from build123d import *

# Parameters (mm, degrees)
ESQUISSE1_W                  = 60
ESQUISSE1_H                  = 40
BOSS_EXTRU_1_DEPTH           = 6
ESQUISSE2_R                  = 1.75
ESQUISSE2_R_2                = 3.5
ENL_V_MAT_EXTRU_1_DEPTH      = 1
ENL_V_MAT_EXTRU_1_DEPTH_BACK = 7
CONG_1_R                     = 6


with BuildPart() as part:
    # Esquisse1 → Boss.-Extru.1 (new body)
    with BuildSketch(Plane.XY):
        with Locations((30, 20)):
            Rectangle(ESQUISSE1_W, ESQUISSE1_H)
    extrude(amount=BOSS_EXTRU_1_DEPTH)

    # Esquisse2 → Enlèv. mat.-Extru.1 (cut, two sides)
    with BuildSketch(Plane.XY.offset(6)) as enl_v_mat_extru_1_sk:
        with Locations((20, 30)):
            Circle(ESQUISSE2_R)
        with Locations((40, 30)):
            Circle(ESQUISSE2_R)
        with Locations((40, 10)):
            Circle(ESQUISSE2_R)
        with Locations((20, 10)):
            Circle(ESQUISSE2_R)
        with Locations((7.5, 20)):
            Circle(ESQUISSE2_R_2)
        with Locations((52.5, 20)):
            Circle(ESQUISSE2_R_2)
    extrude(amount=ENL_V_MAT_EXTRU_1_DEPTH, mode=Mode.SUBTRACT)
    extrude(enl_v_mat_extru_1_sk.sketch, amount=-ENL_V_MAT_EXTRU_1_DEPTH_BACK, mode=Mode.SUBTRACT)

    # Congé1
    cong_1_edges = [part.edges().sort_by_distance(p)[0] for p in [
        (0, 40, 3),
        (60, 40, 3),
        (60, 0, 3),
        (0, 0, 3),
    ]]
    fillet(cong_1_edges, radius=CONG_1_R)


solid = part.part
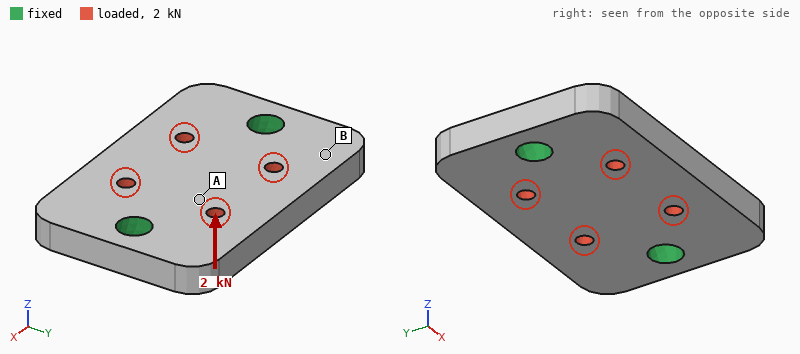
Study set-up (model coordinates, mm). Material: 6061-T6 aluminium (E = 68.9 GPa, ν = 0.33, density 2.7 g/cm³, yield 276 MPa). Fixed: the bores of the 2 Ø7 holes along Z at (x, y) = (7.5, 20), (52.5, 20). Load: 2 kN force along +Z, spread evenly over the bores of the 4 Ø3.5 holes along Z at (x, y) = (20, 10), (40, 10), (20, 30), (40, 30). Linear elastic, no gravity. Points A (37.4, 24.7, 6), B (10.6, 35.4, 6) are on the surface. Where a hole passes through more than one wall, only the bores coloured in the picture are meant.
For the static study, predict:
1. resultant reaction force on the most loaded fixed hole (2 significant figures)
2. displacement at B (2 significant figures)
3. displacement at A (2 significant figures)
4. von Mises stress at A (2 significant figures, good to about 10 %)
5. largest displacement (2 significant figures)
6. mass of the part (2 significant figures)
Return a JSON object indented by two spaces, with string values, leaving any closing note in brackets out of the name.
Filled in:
{
  "resultant reaction force on the most loaded fixed hole": "1.0 kN",
  "displacement at B": "9.2 µm",
  "displacement at A": "14 µm",
  "von Mises stress at A": "22 MPa",
  "largest displacement": "24 µm",
  "mass of the part": "37 g"
}
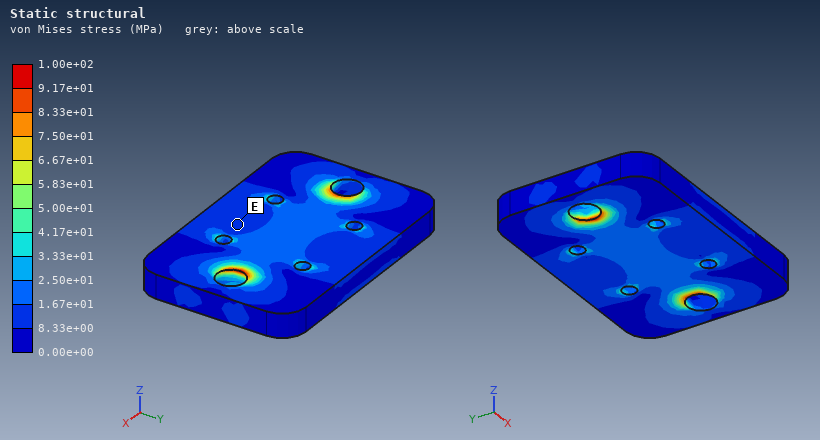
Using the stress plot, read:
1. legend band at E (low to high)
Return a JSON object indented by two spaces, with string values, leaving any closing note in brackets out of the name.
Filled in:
{
  "legend band at E": "8.33e+00 to 1.67e+01 MPa"
}
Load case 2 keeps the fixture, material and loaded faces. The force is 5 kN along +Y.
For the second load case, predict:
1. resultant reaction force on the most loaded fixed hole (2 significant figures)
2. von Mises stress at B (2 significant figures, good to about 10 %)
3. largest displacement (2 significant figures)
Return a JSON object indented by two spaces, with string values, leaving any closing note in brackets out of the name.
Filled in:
{
  "resultant reaction force on the most loaded fixed hole": "2.5 kN",
  "von Mises stress at B": "7.3 MPa",
  "largest displacement": "9.0 µm"
}
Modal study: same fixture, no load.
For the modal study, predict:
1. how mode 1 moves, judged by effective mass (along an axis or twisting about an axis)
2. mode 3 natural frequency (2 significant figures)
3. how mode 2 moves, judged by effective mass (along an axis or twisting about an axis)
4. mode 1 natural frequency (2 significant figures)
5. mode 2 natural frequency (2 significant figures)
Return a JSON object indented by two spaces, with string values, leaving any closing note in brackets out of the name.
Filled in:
{
  "how mode 1 moves, judged by effective mass": "twisting about X",
  "mode 3 natural frequency": "16 kHz",
  "how mode 2 moves, judged by effective mass": "along Z",
  "mode 1 natural frequency": "9200 Hz",
  "mode 2 natural frequency": "11 kHz"
}
